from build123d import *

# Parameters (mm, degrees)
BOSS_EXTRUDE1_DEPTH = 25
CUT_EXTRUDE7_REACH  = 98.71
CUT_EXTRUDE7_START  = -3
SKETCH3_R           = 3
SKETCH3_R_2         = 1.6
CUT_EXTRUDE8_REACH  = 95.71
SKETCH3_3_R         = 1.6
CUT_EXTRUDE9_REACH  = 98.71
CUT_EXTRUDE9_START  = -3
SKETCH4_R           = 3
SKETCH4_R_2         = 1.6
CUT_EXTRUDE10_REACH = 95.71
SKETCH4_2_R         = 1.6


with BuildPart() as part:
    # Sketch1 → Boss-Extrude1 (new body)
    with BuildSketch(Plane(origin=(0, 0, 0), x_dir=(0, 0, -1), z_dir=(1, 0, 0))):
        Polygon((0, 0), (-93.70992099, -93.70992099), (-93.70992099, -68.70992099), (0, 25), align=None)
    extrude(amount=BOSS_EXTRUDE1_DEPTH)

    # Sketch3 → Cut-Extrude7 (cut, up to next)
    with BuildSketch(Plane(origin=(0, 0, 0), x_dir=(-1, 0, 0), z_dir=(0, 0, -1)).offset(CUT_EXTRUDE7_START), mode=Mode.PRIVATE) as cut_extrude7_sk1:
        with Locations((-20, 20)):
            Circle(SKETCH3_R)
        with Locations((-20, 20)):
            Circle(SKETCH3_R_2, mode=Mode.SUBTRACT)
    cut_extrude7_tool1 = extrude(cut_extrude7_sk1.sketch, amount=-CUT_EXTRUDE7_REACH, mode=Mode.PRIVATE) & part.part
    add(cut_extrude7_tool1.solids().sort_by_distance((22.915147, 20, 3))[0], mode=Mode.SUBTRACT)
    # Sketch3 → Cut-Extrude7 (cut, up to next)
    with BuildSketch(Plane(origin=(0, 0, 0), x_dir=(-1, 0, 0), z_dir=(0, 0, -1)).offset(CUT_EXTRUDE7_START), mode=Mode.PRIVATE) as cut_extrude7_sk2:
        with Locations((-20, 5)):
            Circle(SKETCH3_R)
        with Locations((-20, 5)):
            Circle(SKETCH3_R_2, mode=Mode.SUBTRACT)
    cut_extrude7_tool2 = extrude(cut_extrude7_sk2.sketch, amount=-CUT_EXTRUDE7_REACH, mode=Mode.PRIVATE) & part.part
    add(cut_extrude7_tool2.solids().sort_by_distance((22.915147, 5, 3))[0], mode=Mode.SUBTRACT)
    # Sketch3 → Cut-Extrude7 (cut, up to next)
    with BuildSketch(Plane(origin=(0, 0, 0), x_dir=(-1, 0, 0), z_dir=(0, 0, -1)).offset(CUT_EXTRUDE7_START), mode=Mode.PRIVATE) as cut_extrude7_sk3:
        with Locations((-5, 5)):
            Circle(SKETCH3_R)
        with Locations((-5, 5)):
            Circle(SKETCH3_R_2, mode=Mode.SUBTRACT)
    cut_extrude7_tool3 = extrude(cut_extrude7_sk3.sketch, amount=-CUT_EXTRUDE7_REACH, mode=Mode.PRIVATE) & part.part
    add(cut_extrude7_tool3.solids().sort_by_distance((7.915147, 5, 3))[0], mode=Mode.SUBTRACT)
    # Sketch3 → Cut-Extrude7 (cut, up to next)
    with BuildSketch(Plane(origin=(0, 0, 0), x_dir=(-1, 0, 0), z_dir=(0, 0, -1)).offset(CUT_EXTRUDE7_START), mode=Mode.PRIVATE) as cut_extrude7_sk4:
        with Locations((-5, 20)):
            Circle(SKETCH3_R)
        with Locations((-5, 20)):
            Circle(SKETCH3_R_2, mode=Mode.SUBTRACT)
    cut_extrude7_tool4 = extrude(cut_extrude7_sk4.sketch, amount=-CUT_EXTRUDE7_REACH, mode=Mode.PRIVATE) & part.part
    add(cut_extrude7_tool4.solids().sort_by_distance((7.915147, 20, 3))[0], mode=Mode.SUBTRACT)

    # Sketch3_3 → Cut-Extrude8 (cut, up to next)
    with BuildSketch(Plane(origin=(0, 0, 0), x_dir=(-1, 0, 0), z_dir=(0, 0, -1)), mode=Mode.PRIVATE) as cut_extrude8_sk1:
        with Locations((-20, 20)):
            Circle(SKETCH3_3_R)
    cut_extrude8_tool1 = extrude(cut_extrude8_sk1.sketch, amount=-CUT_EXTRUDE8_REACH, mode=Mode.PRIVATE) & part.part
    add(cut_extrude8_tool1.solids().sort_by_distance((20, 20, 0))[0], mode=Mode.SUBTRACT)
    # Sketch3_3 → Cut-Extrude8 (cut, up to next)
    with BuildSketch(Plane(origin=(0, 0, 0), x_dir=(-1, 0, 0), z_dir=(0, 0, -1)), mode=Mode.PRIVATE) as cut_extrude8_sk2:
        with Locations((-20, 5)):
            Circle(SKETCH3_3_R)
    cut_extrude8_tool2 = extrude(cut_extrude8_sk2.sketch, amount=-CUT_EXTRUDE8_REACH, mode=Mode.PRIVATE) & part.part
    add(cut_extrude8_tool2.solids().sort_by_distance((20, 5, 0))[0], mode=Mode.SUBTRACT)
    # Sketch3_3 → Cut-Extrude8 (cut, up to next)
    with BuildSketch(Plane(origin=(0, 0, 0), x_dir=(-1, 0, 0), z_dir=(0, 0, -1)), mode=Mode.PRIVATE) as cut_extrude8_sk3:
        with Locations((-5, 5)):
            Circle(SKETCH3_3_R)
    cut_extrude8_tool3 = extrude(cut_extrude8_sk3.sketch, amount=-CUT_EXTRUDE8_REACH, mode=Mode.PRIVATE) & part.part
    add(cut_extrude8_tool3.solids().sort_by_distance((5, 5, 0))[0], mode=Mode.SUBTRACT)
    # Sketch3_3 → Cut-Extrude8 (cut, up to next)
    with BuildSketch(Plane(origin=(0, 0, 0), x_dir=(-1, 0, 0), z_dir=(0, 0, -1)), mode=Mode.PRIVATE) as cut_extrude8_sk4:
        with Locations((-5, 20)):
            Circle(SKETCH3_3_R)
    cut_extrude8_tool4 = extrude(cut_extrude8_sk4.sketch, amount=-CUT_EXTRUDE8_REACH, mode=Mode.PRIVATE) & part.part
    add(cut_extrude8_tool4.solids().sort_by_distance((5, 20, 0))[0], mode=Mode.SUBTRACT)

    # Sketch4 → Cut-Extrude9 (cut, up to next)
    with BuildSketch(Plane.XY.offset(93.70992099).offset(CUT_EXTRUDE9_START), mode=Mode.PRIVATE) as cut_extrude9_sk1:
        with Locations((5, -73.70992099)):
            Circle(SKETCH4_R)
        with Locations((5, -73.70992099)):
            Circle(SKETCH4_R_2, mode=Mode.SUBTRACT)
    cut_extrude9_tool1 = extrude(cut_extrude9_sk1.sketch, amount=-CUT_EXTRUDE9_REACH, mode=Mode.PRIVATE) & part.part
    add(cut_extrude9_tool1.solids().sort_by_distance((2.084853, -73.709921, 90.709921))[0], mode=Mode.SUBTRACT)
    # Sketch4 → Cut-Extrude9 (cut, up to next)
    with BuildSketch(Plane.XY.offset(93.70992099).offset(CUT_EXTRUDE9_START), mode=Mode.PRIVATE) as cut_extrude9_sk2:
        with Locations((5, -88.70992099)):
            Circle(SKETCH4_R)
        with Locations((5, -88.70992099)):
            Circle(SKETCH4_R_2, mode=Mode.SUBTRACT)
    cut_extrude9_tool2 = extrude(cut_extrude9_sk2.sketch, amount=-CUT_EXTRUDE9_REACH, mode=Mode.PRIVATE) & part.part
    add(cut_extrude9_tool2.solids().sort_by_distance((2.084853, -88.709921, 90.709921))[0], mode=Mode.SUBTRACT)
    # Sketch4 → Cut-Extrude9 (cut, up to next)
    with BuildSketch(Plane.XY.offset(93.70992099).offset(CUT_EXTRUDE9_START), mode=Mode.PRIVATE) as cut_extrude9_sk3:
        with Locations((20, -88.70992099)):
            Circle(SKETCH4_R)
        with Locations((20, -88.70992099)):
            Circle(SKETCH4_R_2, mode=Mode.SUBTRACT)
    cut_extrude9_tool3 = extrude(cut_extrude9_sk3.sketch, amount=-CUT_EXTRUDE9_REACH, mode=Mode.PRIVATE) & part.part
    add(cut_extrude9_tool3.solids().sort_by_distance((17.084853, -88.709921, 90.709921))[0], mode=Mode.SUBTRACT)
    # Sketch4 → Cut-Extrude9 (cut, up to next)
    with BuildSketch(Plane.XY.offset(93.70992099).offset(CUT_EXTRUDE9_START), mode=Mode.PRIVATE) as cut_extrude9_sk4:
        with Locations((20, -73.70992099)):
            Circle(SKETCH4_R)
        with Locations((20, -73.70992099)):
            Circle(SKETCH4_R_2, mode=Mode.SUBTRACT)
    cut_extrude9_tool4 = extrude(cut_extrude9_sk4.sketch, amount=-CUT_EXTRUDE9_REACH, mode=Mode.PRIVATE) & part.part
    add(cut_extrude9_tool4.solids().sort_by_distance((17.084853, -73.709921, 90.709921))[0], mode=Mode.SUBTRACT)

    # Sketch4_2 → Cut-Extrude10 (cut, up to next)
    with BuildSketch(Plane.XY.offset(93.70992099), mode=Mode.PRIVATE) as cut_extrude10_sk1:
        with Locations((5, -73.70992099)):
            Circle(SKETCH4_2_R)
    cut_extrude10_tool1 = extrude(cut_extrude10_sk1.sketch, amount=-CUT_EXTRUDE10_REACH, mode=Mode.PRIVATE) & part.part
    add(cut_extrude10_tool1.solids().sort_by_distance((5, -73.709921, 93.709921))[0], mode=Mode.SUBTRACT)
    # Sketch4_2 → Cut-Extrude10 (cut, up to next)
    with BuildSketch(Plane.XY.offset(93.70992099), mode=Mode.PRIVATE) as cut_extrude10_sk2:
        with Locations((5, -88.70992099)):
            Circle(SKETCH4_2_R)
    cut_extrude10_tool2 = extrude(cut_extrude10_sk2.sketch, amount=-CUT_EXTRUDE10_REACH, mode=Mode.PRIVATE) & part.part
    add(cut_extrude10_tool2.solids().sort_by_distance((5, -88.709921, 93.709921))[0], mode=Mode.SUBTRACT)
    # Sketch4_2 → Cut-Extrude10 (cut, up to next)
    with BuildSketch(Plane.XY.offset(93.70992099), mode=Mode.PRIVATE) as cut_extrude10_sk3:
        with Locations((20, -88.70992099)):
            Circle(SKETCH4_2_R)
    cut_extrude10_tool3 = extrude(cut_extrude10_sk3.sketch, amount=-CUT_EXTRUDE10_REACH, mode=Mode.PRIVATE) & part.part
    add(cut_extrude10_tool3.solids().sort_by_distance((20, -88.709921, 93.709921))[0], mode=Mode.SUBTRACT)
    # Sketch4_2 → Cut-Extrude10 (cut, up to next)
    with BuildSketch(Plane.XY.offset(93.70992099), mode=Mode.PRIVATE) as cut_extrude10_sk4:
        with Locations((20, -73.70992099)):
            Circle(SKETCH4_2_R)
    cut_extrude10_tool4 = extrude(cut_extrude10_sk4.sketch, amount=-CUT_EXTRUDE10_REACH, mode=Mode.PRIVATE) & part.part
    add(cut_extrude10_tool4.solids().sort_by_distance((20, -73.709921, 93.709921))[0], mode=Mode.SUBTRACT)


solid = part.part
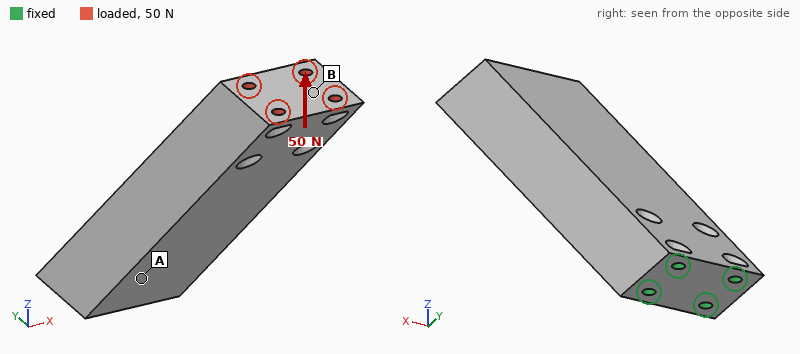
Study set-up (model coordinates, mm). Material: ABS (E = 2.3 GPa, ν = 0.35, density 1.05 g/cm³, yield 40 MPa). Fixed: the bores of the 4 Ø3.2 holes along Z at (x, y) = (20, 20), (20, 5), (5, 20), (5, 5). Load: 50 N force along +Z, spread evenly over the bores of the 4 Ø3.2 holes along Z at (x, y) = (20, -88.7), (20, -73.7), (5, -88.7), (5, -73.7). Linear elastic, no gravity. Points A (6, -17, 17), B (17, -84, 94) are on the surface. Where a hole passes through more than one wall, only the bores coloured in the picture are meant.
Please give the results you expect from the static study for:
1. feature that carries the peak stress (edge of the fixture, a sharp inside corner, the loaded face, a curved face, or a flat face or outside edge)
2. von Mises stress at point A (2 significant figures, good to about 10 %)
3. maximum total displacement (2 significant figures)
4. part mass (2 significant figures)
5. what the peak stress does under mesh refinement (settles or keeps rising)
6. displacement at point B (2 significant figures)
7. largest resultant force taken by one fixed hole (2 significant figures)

edge of the fixture
2.8 MPa
1.5 mm
59 g
keeps rising
1.4 mm
180 N
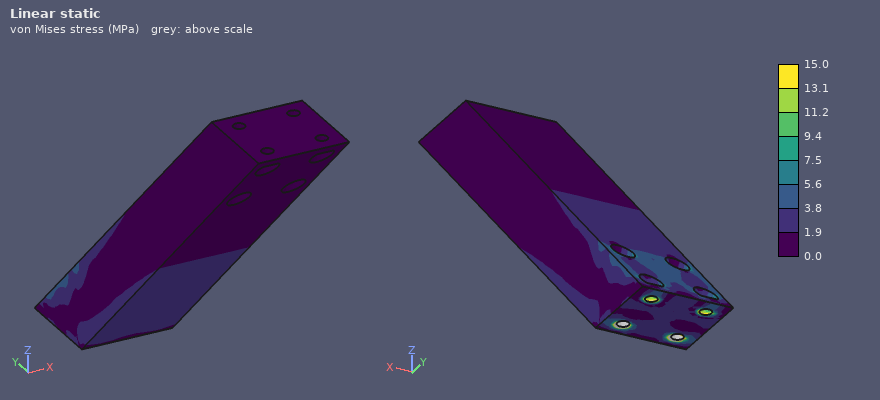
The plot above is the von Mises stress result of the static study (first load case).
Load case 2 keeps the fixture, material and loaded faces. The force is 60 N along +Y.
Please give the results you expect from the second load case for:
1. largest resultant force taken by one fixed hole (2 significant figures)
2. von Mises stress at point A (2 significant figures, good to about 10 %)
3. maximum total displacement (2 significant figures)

200 N
3.1 MPa
1.8 mm
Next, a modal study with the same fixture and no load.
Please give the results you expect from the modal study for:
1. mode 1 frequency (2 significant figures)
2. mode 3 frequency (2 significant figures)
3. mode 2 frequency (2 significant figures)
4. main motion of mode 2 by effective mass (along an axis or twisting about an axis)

200 Hz
1300 Hz
290 Hz
along X
